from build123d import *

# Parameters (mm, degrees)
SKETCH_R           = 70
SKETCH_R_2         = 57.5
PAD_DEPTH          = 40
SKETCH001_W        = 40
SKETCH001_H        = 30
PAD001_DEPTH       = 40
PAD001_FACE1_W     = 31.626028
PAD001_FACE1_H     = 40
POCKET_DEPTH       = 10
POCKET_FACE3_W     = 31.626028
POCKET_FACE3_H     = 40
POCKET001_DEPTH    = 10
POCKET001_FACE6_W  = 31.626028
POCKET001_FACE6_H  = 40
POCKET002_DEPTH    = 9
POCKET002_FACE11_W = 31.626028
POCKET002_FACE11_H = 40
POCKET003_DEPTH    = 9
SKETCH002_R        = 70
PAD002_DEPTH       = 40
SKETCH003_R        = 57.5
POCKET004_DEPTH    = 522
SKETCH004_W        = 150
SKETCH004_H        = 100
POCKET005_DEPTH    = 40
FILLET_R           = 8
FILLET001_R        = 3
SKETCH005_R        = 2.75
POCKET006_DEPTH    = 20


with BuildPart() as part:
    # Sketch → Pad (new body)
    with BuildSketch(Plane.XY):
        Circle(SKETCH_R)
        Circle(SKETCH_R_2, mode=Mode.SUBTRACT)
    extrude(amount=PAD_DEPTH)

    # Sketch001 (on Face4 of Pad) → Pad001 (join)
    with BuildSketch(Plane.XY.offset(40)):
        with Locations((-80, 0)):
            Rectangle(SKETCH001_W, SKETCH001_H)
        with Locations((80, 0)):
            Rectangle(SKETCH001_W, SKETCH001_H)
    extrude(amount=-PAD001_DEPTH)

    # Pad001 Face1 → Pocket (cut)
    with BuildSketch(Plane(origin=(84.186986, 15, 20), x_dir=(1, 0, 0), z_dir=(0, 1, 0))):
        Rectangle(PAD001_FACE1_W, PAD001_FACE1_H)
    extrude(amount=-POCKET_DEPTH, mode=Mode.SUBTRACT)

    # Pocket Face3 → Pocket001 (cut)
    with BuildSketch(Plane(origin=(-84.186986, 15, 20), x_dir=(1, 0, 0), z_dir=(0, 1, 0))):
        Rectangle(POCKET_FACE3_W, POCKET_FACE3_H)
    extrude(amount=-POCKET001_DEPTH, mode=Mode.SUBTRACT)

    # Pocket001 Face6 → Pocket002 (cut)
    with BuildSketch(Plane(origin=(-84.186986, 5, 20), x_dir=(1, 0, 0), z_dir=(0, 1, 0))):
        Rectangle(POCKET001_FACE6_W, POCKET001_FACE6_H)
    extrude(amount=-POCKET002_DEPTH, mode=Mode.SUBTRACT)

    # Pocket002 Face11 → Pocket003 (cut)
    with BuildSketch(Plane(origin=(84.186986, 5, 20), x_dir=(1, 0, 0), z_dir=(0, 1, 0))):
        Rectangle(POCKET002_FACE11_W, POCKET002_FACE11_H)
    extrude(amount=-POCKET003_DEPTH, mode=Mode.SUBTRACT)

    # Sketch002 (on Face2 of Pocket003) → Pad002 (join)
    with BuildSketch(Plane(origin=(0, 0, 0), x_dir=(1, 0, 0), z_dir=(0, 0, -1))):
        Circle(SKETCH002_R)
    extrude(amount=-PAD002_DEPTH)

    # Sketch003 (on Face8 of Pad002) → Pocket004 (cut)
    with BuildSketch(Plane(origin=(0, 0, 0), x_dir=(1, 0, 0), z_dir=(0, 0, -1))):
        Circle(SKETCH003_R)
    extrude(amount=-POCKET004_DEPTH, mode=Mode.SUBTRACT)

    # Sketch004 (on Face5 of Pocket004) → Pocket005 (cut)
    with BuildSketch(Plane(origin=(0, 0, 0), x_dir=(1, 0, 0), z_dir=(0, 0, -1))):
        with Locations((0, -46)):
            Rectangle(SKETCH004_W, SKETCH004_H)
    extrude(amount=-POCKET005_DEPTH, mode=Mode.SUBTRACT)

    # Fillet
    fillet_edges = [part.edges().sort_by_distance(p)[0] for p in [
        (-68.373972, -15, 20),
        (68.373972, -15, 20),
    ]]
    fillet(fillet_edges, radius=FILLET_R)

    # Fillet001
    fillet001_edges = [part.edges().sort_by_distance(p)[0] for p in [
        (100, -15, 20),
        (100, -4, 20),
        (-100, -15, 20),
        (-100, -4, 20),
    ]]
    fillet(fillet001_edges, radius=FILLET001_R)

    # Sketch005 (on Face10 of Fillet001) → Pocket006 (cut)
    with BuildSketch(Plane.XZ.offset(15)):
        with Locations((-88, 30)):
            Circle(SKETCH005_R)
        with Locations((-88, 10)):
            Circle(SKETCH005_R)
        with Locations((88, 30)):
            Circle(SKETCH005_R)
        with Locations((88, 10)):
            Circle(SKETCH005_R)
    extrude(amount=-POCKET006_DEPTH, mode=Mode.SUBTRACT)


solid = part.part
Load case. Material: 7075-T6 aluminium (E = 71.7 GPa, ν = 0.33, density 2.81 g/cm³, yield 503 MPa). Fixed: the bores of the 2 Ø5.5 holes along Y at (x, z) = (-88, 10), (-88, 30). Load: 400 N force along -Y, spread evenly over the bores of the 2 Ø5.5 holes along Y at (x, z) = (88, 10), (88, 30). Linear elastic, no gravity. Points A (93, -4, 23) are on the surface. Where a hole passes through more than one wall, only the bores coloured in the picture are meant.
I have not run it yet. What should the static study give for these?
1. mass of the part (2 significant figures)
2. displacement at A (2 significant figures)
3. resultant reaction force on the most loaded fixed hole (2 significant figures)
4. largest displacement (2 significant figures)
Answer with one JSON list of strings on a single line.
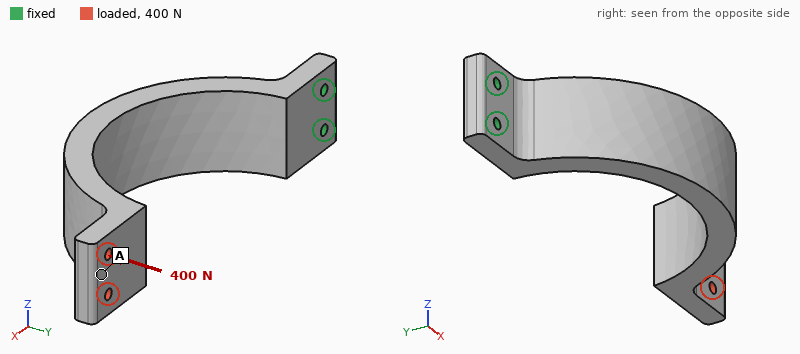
["340 g", "2.3 mm", "270 N", "2.4 mm"]
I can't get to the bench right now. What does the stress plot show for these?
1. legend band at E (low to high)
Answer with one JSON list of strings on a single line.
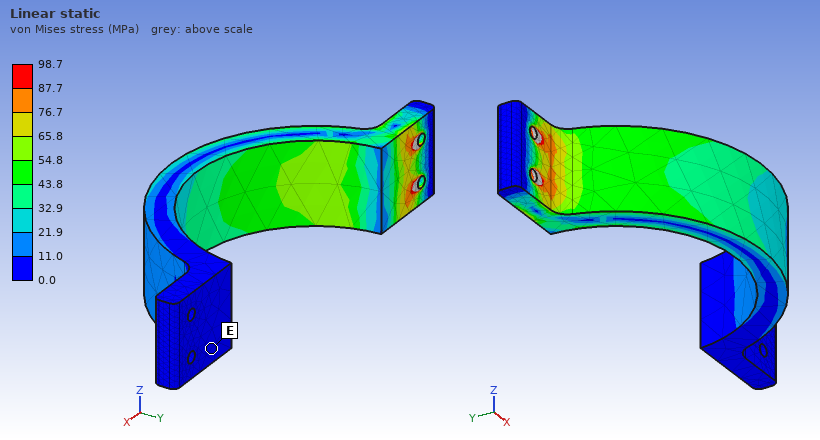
["0.0 to 11.0 MPa"]
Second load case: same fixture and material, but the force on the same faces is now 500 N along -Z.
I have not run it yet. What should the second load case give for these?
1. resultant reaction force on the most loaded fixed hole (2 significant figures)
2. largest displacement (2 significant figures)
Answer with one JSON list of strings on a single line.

["3.8 kN", "1.2 mm"]
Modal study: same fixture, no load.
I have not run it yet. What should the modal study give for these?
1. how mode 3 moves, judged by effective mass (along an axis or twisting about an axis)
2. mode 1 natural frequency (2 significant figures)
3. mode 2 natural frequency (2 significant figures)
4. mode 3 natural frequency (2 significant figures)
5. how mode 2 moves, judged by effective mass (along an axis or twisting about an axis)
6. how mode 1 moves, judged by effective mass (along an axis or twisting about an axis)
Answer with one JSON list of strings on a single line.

["along X", "220 Hz", "370 Hz", "730 Hz", "along Z", "along Y"]
